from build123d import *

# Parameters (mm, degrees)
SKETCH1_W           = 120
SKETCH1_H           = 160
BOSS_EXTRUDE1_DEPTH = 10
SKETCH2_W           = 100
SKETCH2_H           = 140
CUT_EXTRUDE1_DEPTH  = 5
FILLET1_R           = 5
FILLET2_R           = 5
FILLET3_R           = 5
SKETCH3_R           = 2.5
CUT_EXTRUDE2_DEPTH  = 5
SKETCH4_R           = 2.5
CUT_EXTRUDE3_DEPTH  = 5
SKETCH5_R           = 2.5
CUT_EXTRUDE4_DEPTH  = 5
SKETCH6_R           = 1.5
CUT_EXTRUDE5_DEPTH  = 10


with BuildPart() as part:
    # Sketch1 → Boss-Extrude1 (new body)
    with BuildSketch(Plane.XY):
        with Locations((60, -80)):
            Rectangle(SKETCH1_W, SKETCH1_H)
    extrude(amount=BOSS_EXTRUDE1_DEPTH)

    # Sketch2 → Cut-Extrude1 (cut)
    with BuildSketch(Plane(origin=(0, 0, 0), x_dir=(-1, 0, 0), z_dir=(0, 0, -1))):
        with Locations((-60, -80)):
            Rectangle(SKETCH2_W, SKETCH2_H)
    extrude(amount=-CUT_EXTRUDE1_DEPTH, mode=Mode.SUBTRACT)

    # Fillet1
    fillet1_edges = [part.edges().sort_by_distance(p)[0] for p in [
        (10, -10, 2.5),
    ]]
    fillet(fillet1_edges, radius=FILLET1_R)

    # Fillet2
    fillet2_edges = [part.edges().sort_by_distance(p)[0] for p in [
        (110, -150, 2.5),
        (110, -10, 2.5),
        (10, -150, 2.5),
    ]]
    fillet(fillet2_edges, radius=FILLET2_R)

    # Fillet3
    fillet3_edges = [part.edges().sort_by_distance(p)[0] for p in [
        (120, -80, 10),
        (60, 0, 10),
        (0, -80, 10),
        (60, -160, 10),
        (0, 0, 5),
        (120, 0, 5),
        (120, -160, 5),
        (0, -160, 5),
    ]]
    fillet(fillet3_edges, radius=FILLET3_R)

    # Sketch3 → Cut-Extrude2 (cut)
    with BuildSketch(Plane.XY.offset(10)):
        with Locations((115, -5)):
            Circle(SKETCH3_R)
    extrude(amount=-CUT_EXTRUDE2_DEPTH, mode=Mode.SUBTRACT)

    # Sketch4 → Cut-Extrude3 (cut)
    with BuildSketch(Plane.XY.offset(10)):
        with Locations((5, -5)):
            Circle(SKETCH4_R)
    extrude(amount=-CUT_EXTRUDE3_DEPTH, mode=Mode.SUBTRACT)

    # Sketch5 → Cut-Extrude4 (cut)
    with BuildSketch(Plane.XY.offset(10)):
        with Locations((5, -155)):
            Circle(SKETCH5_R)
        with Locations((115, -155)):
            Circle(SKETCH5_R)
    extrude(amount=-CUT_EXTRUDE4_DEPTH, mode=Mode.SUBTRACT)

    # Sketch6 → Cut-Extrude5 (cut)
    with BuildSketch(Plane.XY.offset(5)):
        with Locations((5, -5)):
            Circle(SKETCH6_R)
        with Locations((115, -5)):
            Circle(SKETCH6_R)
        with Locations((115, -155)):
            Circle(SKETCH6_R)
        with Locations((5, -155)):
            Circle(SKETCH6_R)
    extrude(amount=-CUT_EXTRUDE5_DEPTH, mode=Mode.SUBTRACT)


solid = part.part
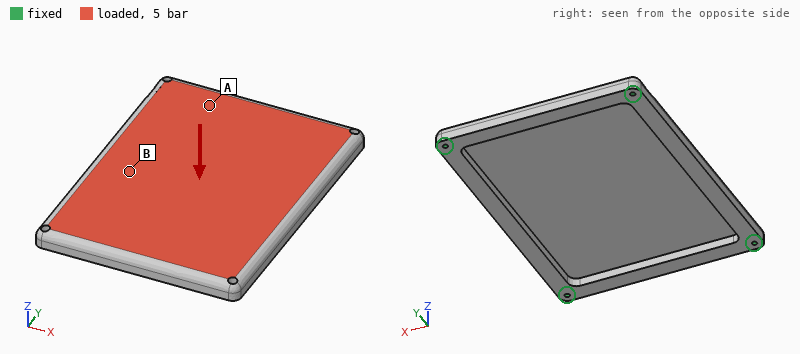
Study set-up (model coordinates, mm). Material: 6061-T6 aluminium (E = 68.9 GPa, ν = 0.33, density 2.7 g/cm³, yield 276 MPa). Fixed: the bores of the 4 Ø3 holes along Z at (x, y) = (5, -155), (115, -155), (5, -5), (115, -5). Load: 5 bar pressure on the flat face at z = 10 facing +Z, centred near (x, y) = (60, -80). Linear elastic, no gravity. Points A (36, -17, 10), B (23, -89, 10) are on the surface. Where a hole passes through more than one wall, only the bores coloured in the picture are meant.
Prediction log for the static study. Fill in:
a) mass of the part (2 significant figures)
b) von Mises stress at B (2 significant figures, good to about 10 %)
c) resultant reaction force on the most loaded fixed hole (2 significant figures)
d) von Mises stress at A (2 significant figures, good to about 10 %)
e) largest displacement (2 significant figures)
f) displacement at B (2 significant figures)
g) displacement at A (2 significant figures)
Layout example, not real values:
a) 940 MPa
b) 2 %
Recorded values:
a) 320 g
b) 78 MPa
c) 6.3 kN
d) 35 MPa
e) 0.82 mm
f) 0.62 mm
g) 0.24 mm
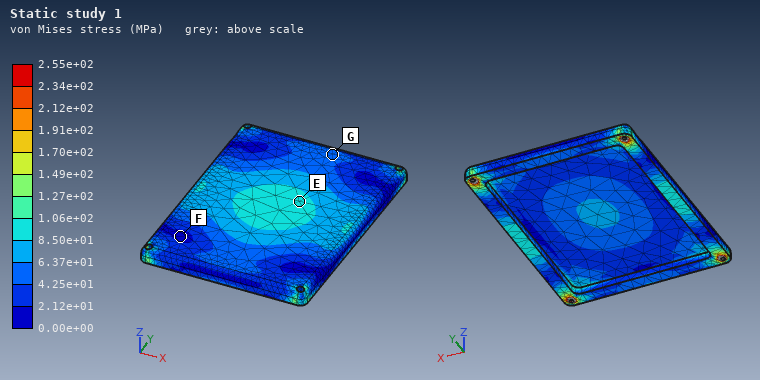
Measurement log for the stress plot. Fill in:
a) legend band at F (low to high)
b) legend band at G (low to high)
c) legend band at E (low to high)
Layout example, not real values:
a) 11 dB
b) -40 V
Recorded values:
a) 0.00e+00 to 2.12e+01 MPa
b) 4.25e+01 to 6.37e+01 MPa
c) 8.50e+01 to 1.06e+02 MPa
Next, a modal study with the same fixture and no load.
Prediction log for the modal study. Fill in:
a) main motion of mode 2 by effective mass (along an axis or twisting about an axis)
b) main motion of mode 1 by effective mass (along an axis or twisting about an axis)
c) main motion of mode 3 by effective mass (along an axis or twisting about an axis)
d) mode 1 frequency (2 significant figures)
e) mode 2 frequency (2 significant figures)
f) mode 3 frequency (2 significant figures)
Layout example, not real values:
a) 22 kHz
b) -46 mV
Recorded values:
a) twisting about Y
b) along Z
c) twisting about X
d) 1200 Hz
e) 1800 Hz
f) 2500 Hz
